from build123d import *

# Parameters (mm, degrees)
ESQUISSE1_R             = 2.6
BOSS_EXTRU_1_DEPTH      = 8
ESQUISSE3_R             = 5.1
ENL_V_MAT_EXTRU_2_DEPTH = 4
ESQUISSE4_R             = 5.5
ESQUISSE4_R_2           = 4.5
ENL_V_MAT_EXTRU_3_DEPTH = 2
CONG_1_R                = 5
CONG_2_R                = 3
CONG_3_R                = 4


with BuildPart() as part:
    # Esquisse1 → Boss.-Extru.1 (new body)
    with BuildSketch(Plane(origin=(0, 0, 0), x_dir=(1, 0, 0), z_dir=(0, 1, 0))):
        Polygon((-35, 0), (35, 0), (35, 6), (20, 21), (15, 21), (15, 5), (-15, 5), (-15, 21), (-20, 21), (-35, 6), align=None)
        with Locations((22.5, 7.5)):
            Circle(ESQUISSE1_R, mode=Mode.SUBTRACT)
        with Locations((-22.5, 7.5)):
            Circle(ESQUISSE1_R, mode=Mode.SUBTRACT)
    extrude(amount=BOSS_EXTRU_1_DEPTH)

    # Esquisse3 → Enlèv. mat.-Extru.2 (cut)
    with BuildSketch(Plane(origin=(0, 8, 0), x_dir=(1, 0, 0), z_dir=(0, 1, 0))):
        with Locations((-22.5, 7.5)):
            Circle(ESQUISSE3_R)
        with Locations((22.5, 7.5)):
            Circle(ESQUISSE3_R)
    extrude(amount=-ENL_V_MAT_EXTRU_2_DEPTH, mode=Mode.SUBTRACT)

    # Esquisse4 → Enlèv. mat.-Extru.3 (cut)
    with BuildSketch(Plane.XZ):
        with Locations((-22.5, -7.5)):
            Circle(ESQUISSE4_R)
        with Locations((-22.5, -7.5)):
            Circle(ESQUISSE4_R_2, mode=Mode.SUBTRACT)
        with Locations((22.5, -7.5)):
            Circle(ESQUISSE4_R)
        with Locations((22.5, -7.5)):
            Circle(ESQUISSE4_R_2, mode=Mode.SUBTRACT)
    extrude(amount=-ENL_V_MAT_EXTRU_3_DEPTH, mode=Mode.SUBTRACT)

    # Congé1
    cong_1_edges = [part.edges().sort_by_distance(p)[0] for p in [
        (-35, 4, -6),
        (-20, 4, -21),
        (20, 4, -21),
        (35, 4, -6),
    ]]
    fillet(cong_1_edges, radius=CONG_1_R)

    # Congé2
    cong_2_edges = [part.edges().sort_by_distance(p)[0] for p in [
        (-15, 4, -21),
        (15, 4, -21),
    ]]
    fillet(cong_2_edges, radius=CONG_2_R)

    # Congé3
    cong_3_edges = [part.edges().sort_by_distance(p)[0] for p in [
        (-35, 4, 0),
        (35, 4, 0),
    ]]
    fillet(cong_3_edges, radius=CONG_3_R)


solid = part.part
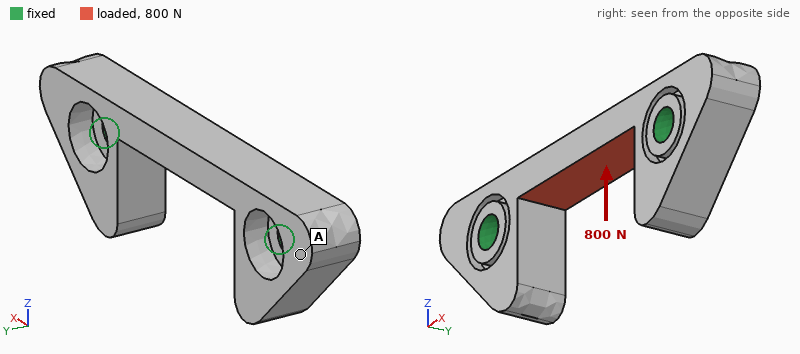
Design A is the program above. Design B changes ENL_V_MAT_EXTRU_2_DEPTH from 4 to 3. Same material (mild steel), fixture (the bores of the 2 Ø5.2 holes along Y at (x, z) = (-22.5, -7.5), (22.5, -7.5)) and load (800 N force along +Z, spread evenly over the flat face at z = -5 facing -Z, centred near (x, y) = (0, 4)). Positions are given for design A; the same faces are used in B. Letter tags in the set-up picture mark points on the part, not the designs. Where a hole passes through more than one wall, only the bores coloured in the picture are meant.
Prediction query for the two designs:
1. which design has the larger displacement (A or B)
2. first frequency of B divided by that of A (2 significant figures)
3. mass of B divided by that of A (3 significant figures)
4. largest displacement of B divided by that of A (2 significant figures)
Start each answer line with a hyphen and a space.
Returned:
- A
- 1.1
- 1.02
- 0.90
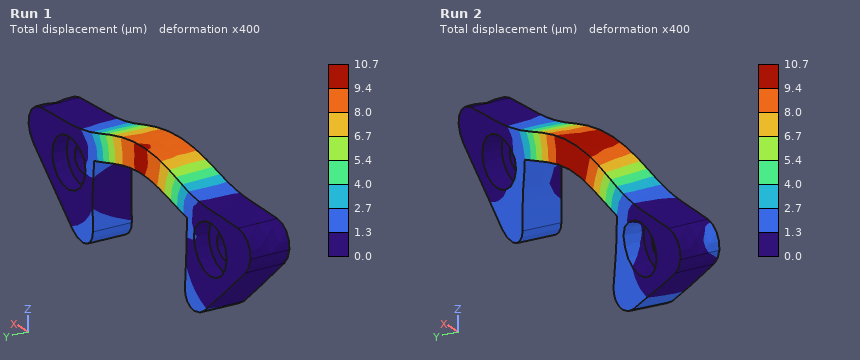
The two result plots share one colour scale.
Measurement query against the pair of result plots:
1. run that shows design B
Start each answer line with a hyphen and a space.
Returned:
- Run 1
